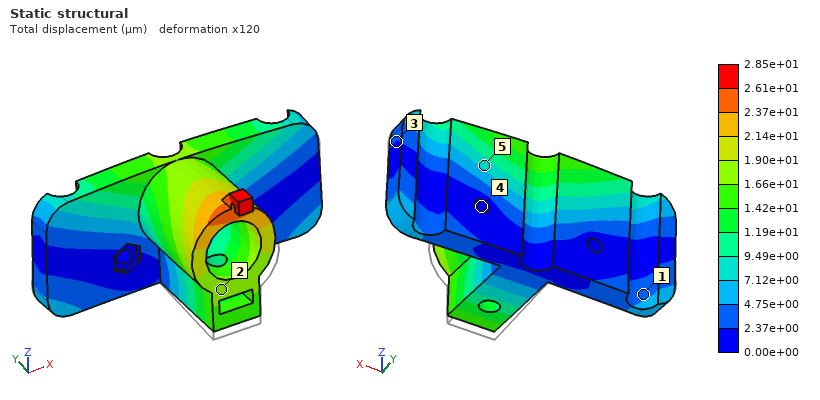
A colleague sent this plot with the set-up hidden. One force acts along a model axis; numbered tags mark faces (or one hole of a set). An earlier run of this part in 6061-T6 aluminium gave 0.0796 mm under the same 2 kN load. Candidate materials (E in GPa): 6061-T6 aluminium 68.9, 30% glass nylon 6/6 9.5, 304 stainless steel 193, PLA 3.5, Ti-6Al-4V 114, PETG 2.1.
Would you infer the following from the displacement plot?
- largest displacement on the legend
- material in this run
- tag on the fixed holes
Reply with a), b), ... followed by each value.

a) 2.85e+01 µm
b) 304 stainless steel
c) 4
